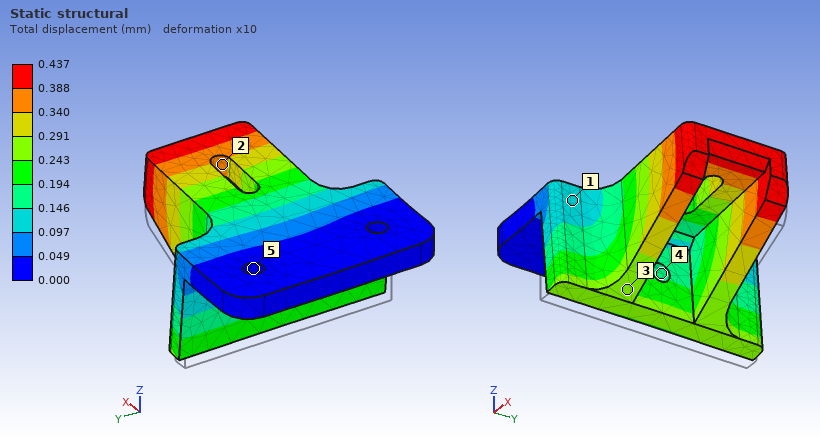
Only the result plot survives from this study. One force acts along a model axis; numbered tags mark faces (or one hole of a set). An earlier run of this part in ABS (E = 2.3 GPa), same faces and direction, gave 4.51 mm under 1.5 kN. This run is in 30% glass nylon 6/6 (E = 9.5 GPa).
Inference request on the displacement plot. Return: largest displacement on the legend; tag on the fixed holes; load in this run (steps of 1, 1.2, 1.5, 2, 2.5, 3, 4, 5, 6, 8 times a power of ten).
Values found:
0.437 mm
5
600 N
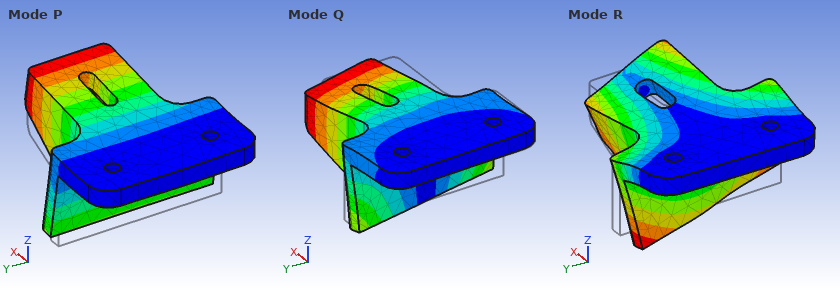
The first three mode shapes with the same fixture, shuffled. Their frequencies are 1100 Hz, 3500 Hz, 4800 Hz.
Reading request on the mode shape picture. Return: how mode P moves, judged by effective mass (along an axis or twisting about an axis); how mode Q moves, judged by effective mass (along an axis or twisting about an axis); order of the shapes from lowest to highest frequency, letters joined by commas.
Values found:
along Z
along Y
P, R, Q
